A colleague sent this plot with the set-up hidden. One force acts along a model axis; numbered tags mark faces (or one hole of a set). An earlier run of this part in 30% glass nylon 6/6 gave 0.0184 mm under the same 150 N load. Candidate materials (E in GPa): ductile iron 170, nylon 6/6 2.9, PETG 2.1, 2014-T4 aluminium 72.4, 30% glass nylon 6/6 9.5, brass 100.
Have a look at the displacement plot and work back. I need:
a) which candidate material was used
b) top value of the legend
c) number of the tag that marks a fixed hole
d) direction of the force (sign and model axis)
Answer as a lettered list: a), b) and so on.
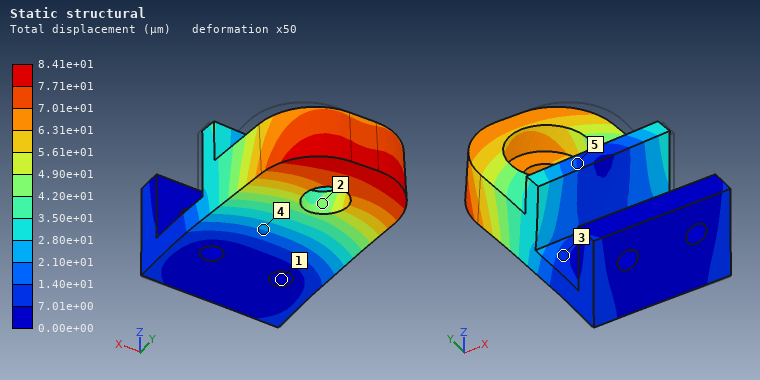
a) PETG
b) 8.41e+01 µm
c) 1
d) -X
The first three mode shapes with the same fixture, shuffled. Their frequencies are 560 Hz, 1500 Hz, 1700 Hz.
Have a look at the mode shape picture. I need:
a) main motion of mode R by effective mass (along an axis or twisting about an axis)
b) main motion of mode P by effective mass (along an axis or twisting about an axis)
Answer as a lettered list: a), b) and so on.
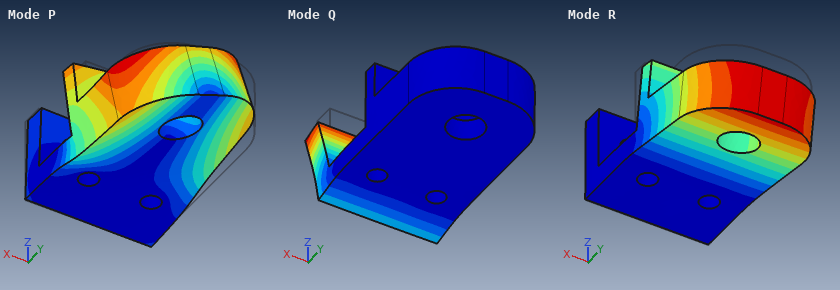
a) along Z
b) along X
